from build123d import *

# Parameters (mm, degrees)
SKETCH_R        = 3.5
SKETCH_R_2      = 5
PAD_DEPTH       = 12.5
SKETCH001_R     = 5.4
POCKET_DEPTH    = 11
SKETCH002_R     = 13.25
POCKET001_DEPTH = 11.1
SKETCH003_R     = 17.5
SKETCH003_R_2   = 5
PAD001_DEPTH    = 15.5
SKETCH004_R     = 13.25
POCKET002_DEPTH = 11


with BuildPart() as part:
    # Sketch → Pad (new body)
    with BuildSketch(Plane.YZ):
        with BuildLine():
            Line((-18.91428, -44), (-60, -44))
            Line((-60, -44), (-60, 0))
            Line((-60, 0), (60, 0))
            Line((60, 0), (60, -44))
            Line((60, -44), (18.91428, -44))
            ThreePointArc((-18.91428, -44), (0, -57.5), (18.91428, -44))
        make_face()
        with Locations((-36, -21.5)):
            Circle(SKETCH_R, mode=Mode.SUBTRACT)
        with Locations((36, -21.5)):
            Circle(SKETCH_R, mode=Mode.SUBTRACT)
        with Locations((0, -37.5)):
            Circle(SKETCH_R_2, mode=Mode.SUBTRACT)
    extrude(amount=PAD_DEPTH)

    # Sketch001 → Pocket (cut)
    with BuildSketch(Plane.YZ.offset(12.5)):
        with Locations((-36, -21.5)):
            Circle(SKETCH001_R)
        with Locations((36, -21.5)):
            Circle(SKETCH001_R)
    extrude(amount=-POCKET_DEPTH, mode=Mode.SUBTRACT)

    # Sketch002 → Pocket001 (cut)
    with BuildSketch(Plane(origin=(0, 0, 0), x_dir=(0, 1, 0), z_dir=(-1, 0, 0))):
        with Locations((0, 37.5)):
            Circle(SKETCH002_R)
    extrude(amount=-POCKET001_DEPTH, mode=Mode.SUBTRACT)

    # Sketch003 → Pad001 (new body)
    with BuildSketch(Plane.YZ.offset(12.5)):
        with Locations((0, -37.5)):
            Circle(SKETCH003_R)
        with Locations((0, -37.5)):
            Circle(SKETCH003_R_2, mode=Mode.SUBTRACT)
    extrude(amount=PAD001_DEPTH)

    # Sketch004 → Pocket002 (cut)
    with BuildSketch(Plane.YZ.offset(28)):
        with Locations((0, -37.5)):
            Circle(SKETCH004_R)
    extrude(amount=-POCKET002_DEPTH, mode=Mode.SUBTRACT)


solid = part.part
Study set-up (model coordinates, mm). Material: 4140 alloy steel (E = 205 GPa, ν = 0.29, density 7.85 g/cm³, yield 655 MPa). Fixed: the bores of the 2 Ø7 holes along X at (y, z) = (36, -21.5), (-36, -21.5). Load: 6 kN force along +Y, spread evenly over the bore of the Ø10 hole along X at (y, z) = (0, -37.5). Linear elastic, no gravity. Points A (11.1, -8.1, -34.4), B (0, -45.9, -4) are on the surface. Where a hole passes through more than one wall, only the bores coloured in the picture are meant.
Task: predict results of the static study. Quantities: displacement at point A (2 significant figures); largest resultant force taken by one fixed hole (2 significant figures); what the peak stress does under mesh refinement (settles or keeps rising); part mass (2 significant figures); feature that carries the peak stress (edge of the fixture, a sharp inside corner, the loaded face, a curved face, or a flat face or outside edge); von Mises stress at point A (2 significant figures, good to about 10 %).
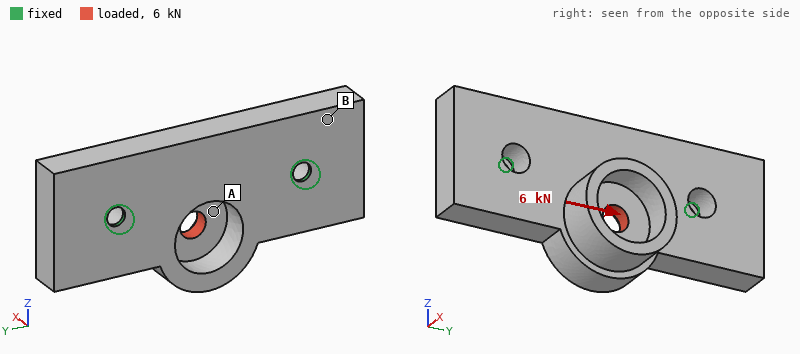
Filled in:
6.0 µm
3.5 kN
keeps rising
560 g
edge of the fixture
33 MPa
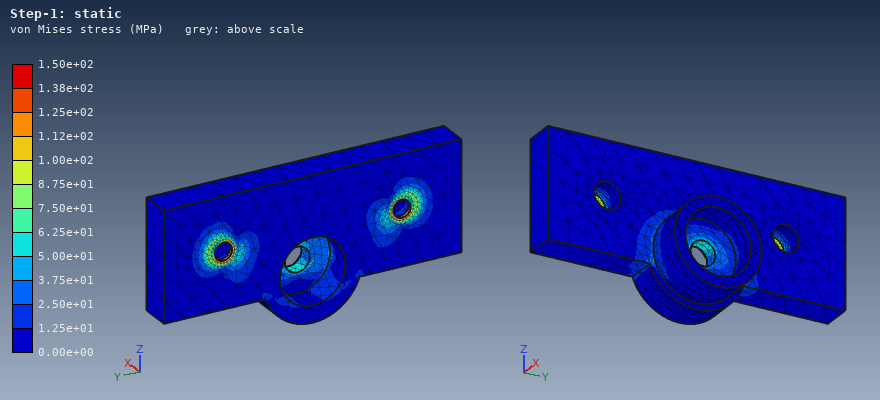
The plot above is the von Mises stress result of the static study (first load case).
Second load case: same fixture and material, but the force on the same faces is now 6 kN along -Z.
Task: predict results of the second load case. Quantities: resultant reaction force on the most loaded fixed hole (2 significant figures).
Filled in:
3.0 kN
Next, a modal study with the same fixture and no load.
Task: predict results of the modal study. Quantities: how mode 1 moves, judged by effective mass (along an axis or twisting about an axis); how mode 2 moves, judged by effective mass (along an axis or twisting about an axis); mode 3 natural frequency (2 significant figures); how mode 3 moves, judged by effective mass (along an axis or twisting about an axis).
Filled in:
along Z
along X
5900 Hz
twisting about X
